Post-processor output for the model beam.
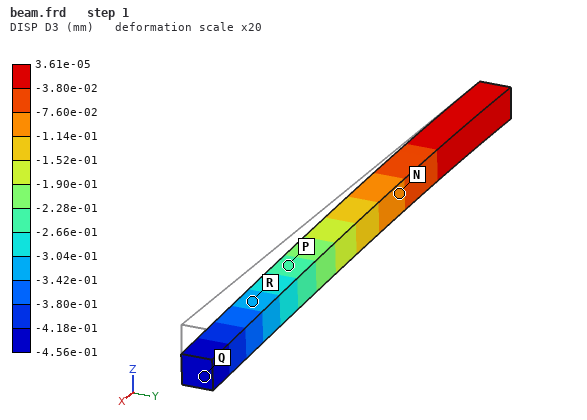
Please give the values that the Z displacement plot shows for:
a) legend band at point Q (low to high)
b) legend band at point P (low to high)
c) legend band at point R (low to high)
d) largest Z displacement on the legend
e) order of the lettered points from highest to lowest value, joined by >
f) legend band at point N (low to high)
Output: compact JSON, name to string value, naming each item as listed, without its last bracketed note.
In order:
{"legend band at point Q": "-4.56e-01 to -4.18e-01 mm", "legend band at point P": "-2.66e-01 to -2.28e-01 mm", "legend band at point R": "-3.42e-01 to -3.04e-01 mm", "largest Z displacement on the legend": "3.61e-05 mm", "order of the lettered points from highest to lowest value, joined by >": "N > P > R > Q", "legend band at point N": "-1.14e-01 to -7.60e-02 mm"}
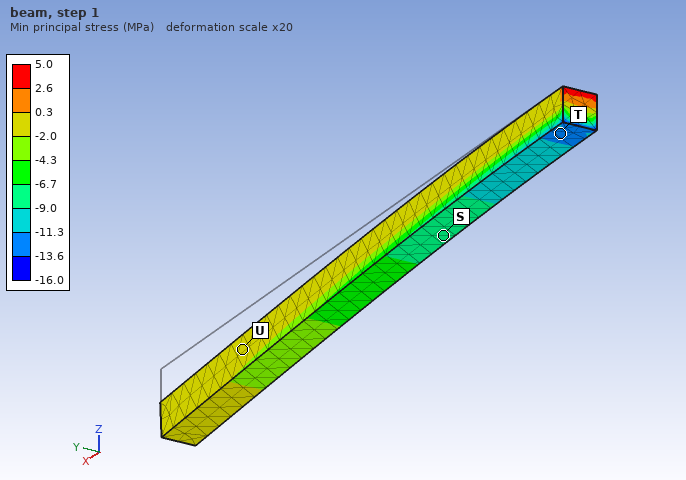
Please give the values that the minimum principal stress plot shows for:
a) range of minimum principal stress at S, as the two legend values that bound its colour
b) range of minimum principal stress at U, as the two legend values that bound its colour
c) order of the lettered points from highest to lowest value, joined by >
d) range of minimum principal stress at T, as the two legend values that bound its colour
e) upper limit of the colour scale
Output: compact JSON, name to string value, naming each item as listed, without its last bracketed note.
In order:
{"range of minimum principal stress at S, as the two legend values that bound its colour": "-9.0 to -6.7 MPa", "range of minimum principal stress at U, as the two legend values that bound its colour": "-2.0 to 0.3 MPa", "order of the lettered points from highest to lowest value, joined by >": "U > S > T", "range of minimum principal stress at T, as the two legend values that bound its colour": "-13.6 to -11.3 MPa", "upper limit of the colour scale": "5.0 MPa"}
